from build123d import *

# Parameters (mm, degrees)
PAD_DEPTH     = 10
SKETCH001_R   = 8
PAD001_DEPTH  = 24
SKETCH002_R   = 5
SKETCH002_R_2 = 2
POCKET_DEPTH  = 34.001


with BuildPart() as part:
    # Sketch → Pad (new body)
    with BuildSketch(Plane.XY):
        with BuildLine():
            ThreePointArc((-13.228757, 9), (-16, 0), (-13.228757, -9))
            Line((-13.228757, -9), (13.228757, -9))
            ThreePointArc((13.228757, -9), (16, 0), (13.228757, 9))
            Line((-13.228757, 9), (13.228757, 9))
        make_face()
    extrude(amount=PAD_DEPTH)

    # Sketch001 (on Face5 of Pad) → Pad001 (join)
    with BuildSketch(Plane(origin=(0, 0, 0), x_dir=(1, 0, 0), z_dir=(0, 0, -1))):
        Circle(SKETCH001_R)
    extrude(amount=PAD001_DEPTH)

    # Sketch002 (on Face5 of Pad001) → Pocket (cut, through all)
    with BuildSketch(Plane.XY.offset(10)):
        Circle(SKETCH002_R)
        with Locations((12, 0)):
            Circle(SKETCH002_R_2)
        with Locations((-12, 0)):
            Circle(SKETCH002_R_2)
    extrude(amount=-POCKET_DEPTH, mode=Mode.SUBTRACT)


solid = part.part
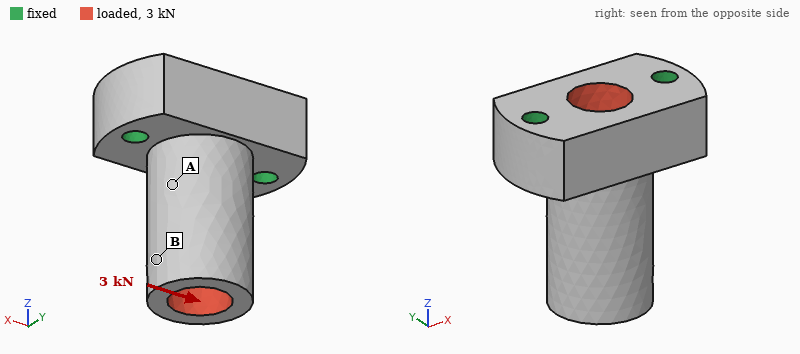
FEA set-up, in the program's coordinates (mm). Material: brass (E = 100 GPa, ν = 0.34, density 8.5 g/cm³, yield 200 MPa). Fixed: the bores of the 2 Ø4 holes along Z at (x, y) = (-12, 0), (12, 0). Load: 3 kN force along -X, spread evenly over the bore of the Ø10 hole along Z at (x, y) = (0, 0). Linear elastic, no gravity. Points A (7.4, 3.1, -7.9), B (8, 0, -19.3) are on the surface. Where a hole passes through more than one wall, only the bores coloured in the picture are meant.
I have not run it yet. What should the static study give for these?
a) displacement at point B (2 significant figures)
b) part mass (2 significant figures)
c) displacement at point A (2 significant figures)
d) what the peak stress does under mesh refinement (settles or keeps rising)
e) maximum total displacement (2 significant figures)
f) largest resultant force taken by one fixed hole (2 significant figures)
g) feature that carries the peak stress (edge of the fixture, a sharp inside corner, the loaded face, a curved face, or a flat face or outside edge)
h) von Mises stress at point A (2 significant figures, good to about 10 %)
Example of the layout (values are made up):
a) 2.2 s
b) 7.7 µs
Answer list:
a) 29 µm
b) 62 g
c) 14 µm
d) keeps rising
e) 35 µm
f) 2.3 kN
g) a sharp inside corner
h) 29 MPa
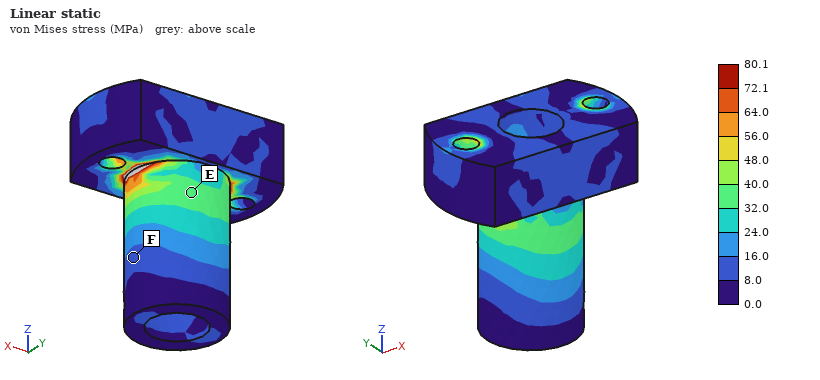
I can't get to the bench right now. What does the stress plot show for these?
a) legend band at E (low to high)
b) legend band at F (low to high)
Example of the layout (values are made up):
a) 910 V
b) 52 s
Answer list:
a) 32.0 to 40.0 MPa
b) 8.0 to 16.0 MPa
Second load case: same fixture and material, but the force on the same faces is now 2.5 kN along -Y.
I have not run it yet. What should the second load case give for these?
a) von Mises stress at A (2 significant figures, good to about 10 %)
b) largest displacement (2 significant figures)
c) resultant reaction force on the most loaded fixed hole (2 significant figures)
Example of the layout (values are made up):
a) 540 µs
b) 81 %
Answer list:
a) 25 MPa
b) 53 µm
c) 1.3 kN
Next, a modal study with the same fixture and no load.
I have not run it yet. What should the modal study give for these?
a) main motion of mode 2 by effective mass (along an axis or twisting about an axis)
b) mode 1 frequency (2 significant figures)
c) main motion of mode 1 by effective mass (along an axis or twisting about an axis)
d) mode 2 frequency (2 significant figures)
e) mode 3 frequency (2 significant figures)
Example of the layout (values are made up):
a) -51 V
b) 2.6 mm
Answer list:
a) along X
b) 6900 Hz
c) along Y
d) 9300 Hz
e) 20 kHz
